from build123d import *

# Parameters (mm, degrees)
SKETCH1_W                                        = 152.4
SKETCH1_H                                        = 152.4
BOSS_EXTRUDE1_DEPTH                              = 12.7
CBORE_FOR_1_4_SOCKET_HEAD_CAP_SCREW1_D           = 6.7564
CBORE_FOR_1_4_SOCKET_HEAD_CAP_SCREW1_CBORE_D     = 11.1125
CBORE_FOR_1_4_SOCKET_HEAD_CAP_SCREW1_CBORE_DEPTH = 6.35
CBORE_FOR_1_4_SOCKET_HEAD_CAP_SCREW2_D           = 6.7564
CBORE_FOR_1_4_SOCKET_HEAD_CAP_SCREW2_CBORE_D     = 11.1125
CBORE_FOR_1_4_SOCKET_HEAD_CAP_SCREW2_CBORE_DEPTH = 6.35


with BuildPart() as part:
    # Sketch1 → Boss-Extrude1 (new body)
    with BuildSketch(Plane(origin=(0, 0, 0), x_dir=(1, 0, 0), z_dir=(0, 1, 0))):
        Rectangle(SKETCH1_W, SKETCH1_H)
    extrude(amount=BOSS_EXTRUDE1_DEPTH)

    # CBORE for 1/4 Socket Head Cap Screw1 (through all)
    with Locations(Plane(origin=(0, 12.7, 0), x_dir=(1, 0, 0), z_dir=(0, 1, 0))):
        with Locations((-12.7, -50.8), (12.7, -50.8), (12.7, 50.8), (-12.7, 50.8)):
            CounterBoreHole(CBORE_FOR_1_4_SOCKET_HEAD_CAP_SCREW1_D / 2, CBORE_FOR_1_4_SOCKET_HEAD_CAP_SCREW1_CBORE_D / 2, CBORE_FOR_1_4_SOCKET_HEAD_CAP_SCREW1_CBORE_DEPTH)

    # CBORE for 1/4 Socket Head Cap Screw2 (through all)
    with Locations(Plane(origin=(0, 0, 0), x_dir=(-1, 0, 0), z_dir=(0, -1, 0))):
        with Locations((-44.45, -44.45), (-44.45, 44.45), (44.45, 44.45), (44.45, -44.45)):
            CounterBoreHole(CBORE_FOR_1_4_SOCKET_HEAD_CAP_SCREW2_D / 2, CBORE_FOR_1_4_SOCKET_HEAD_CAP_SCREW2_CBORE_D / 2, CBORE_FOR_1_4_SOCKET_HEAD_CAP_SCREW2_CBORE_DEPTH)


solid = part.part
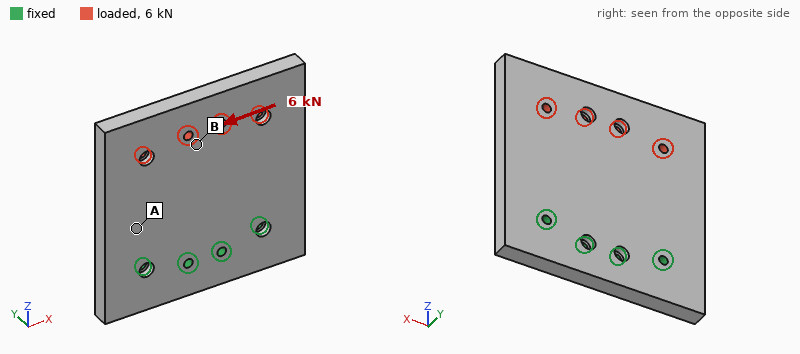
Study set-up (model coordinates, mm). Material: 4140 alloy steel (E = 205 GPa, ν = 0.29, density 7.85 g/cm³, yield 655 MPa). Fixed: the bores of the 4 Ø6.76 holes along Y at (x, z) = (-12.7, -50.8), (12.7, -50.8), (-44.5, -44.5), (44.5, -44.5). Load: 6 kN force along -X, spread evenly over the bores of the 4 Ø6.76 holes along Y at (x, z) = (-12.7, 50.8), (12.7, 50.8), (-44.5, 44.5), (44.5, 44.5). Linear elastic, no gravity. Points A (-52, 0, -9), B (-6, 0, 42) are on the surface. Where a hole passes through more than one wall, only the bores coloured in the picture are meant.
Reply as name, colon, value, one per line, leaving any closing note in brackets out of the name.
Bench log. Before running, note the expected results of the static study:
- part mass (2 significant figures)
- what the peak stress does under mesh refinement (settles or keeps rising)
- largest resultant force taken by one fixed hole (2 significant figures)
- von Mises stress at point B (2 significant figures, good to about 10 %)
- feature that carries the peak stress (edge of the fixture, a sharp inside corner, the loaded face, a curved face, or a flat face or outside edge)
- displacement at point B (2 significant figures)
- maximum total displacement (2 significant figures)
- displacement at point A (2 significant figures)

part mass: 2.3 kg
what the peak stress does under mesh refinement: keeps rising
largest resultant force taken by one fixed hole: 6.1 kN
von Mises stress at point B: 9.2 MPa
feature that carries the peak stress: edge of the fixture
displacement at point B: 10 µm
maximum total displacement: 17 µm
displacement at point A: 6.1 µm
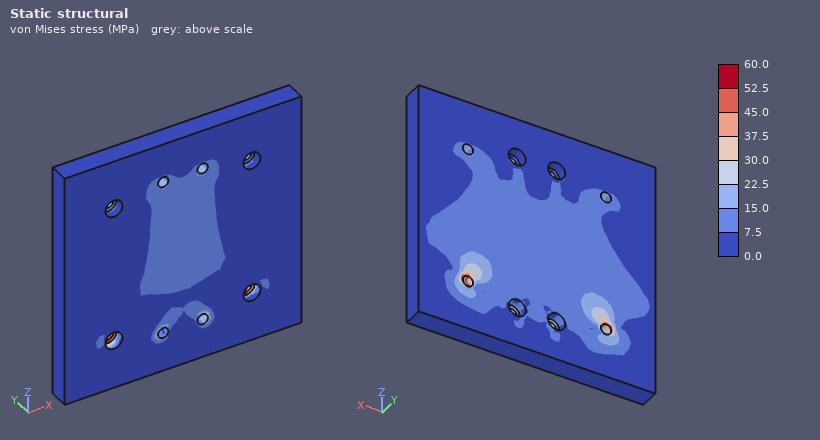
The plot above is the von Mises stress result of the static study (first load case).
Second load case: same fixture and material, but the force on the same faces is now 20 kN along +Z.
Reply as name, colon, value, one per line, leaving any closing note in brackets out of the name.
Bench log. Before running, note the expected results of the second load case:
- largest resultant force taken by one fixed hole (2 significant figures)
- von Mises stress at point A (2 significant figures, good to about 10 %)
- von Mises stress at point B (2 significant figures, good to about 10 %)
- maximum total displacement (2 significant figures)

largest resultant force taken by one fixed hole: 5.8 kN
von Mises stress at point A: 9.5 MPa
von Mises stress at point B: 22 MPa
maximum total displacement: 17 µm
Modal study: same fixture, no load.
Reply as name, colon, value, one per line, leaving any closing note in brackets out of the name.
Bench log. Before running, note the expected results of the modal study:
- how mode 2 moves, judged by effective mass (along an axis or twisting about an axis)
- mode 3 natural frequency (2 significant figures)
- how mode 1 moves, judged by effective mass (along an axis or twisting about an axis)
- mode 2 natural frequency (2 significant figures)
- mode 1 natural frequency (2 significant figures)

how mode 2 moves, judged by effective mass: twisting about Z
mode 3 natural frequency: 3200 Hz
how mode 1 moves, judged by effective mass: along Y
mode 2 natural frequency: 1200 Hz
mode 1 natural frequency: 570 Hz
